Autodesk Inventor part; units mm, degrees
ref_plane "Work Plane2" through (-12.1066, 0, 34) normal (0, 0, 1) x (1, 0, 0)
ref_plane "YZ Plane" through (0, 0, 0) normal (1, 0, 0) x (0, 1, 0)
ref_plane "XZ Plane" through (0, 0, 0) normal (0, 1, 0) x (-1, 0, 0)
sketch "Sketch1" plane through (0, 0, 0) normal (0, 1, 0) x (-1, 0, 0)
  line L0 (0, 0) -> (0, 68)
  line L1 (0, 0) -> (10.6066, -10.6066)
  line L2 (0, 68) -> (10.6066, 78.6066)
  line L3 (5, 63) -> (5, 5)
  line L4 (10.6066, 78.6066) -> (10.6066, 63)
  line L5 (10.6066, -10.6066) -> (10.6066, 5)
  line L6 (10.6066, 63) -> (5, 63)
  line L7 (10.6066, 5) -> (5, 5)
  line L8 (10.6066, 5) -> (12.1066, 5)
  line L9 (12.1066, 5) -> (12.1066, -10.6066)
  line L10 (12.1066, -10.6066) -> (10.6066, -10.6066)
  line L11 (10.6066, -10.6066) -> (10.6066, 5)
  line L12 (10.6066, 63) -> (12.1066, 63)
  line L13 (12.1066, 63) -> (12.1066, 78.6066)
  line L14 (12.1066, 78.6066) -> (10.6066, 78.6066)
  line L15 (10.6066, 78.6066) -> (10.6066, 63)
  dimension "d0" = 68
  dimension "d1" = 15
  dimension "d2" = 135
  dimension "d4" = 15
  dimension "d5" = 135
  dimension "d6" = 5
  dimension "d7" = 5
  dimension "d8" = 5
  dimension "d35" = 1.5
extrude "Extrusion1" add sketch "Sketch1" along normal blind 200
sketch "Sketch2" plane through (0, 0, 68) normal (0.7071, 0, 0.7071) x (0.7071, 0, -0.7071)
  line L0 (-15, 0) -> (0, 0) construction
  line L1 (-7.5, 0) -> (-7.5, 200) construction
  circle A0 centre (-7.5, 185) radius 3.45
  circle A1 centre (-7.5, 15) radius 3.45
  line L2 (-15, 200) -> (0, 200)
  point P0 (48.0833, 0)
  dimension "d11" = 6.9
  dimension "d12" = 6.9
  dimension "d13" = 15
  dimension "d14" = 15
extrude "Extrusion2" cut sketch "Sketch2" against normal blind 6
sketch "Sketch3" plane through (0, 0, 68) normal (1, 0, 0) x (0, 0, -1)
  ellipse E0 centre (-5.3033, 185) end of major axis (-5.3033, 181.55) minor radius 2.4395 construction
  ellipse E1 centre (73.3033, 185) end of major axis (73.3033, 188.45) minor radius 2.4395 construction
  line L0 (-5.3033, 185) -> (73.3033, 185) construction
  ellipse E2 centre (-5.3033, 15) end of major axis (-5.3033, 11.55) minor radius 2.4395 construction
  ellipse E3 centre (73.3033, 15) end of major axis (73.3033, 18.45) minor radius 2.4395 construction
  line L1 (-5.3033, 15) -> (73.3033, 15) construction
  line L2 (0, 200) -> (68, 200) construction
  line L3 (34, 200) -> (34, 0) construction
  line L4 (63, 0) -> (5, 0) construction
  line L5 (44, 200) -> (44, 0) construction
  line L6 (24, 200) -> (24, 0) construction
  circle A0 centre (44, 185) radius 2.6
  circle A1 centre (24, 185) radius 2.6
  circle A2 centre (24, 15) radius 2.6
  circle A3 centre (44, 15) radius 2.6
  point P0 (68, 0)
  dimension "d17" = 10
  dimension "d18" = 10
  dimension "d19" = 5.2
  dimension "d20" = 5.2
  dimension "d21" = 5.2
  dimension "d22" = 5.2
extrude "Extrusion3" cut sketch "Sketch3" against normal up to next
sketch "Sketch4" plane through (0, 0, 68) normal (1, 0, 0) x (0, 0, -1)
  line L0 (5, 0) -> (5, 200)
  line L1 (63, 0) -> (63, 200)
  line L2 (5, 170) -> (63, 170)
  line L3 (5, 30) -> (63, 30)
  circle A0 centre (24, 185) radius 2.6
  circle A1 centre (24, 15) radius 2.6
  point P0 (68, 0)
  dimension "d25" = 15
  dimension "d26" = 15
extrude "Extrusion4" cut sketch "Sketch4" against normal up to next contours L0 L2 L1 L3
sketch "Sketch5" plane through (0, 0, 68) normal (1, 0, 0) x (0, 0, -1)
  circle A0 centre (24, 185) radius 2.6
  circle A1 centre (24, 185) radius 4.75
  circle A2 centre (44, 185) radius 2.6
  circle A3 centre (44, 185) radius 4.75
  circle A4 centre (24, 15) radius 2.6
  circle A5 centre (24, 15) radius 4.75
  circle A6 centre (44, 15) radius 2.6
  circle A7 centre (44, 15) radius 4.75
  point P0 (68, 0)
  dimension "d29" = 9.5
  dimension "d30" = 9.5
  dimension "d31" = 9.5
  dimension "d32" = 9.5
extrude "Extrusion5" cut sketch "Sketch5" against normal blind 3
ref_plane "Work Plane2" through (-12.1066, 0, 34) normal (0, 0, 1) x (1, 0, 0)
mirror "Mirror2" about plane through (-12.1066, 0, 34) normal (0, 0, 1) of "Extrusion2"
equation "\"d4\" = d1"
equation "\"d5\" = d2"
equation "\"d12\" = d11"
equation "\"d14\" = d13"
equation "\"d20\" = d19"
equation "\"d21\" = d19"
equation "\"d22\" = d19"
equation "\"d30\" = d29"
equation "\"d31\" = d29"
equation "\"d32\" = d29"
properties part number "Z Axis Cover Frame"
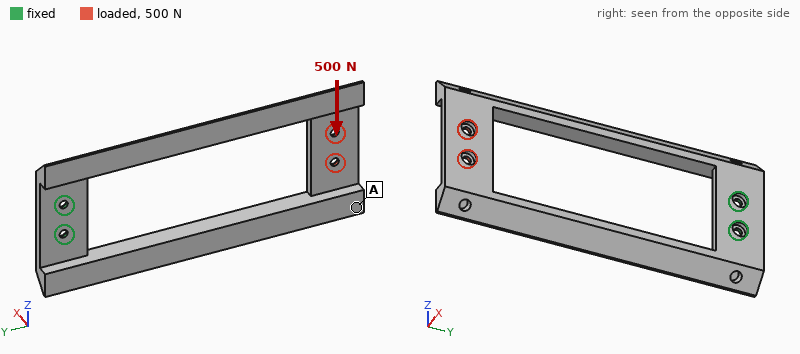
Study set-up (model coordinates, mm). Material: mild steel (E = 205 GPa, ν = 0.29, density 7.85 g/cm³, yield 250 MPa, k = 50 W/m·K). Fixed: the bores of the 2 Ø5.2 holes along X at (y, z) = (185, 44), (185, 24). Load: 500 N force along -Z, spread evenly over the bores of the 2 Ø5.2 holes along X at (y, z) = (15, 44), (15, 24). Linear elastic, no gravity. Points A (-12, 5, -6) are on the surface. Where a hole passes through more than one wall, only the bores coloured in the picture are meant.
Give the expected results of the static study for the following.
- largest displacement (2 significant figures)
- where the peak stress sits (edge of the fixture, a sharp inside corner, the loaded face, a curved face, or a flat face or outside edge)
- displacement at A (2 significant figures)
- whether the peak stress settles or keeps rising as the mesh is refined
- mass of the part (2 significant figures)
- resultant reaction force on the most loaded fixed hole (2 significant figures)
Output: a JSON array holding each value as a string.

["0.41 mm", "edge of the fixture", "0.41 mm", "keeps rising", "540 g", "3.6 kN"]
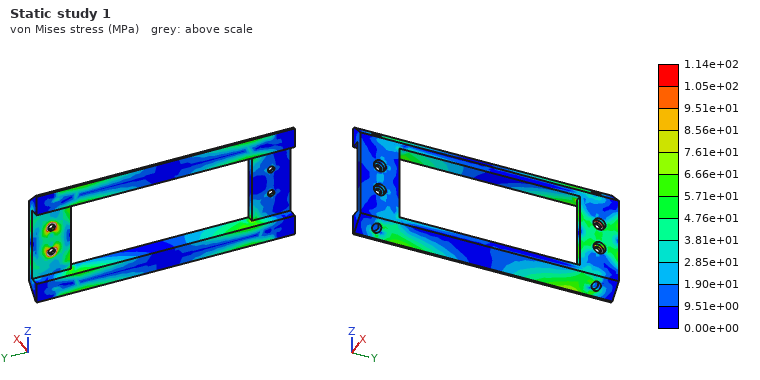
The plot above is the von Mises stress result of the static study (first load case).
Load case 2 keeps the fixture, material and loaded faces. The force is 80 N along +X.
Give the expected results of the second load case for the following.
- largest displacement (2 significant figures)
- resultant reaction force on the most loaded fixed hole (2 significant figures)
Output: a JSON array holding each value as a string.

["0.72 mm", "57 N"]
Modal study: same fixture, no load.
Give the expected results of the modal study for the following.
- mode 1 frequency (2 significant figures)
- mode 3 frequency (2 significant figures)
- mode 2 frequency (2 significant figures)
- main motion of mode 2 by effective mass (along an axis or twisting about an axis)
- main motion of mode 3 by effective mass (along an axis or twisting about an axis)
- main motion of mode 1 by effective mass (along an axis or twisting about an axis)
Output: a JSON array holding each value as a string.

["120 Hz", "430 Hz", "370 Hz", "along Z", "along Z", "along X"]
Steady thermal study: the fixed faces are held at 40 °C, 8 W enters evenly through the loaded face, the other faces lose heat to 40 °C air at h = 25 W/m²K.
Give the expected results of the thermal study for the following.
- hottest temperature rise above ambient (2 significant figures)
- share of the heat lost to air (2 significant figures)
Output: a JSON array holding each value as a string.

["36 K", "93 %"]
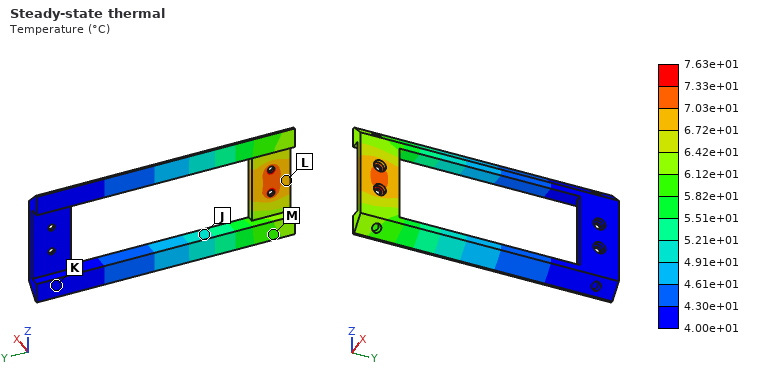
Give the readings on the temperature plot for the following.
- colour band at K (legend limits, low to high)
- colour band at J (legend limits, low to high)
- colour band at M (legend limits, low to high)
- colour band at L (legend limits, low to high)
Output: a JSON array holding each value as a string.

["4.00e+01 to 4.30e+01 °C", "4.91e+01 to 5.21e+01 °C", "5.82e+01 to 6.12e+01 °C", "6.72e+01 to 7.03e+01 °C"]
